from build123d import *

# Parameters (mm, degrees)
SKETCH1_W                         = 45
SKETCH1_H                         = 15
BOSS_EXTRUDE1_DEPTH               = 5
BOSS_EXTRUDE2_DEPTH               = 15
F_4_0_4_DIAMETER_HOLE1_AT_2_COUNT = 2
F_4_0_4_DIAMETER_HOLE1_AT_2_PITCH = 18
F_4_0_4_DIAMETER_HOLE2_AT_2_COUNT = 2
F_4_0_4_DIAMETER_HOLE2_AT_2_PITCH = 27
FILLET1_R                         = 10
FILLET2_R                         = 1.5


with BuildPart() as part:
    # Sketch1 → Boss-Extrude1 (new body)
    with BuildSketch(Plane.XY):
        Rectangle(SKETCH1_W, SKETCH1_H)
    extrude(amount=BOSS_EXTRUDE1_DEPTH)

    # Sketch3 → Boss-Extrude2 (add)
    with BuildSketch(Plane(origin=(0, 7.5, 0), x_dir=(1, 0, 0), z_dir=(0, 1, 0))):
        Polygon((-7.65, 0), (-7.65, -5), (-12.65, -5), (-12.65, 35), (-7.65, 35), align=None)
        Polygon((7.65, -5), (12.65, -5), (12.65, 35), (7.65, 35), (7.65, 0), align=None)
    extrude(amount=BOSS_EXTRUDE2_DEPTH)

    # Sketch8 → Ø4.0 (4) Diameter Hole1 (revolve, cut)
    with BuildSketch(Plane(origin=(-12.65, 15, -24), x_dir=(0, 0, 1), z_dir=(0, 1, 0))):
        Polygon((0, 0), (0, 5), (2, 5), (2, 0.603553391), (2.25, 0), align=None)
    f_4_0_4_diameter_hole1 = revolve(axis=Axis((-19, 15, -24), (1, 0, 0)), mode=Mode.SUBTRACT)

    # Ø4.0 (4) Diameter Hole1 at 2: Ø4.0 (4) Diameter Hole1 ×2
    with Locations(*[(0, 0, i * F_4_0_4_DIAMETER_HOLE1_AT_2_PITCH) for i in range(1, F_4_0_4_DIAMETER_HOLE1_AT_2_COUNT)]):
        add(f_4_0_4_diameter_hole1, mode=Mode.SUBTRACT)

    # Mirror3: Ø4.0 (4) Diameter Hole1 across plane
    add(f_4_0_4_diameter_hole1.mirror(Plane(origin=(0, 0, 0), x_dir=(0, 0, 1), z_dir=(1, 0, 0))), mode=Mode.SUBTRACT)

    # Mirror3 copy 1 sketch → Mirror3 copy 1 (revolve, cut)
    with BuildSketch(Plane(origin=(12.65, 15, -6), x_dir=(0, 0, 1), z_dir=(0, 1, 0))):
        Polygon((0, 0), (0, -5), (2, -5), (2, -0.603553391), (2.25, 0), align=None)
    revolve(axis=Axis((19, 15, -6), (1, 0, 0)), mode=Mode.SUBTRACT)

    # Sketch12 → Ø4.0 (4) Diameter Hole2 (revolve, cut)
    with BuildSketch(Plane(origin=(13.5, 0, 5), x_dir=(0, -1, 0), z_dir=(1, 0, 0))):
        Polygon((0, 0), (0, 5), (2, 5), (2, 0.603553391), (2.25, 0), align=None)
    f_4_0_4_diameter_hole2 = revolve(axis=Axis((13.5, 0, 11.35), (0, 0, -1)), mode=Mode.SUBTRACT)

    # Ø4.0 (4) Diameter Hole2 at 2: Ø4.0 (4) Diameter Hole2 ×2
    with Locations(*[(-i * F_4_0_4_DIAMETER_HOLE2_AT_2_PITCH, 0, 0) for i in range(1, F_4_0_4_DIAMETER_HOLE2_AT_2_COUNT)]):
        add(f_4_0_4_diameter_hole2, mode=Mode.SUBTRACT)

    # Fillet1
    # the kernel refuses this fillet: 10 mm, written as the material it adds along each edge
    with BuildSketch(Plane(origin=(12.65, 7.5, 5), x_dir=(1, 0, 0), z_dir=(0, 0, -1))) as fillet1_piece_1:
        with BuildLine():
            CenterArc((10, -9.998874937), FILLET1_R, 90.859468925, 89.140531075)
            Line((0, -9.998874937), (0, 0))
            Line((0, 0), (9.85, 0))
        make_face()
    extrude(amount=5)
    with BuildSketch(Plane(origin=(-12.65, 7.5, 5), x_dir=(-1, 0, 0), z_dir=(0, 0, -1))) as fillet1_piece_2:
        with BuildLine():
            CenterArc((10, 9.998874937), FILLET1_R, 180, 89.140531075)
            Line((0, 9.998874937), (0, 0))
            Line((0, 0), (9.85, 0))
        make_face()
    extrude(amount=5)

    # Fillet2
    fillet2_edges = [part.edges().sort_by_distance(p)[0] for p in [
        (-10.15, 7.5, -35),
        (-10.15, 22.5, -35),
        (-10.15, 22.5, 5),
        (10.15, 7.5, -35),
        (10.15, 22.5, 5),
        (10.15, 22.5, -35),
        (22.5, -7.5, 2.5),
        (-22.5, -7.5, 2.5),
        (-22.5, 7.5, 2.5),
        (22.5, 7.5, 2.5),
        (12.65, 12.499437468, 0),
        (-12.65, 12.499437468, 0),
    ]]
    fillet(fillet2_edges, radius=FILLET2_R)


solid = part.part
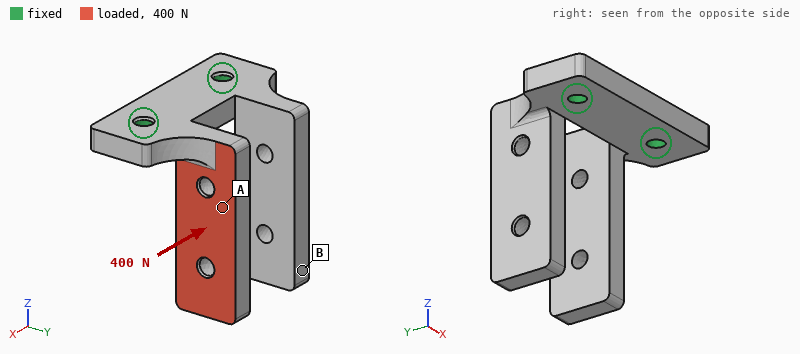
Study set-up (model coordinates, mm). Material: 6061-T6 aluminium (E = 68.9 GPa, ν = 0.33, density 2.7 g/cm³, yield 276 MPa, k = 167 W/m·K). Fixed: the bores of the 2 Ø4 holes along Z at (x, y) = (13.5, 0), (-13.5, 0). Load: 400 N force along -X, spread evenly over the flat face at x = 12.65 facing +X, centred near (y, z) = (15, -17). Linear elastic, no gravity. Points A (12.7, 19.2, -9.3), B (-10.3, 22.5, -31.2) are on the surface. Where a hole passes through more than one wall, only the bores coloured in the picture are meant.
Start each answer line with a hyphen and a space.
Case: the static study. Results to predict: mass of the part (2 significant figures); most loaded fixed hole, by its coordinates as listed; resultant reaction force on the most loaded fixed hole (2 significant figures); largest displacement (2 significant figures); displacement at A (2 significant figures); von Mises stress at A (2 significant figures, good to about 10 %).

- 25 g
- (13.5, 0)
- 380 N
- 0.57 mm
- 0.15 mm
- 64 MPa
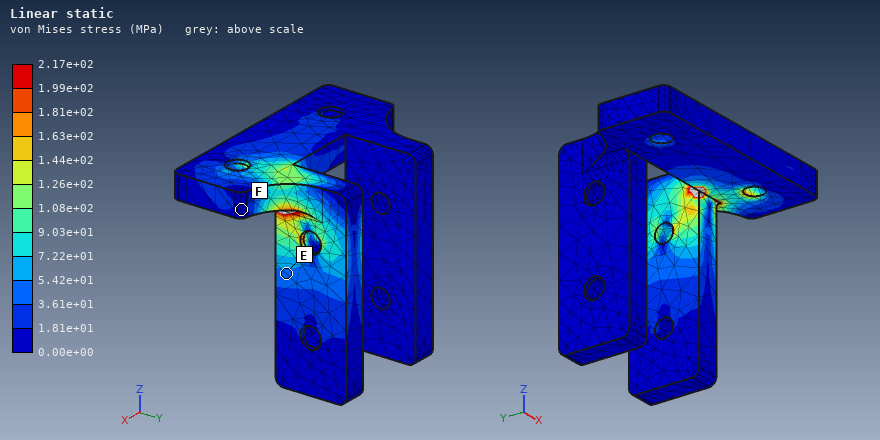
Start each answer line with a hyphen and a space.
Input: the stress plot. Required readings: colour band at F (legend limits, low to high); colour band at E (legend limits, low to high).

- 0.00e+00 to 1.81e+01 MPa
- 3.61e+01 to 5.42e+01 MPa
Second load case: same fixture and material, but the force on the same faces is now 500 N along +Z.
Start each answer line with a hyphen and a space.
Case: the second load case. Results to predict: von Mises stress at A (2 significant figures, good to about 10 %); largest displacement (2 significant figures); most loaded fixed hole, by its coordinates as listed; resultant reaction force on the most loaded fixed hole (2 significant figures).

- 23 MPa
- 0.26 mm
- (13.5, 0)
- 510 N
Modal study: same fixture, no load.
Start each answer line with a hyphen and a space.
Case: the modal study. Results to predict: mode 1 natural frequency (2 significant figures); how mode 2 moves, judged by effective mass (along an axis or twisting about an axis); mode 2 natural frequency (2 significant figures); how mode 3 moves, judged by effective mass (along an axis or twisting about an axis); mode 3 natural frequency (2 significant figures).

- 1900 Hz
- along X
- 2000 Hz
- along Y
- 2100 Hz
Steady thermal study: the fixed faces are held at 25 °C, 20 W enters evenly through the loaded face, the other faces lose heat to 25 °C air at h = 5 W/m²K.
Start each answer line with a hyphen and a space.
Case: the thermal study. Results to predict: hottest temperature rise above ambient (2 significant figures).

- 57 K
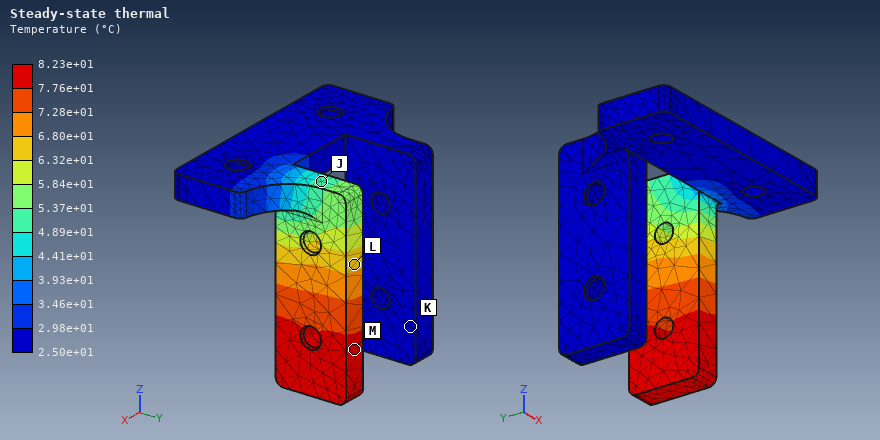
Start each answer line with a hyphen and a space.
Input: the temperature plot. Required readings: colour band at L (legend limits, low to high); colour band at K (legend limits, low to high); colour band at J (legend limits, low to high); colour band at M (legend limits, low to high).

- 6.32e+01 to 6.80e+01 °C
- 2.50e+01 to 2.98e+01 °C
- 4.89e+01 to 5.37e+01 °C
- 7.76e+01 to 8.23e+01 °C
